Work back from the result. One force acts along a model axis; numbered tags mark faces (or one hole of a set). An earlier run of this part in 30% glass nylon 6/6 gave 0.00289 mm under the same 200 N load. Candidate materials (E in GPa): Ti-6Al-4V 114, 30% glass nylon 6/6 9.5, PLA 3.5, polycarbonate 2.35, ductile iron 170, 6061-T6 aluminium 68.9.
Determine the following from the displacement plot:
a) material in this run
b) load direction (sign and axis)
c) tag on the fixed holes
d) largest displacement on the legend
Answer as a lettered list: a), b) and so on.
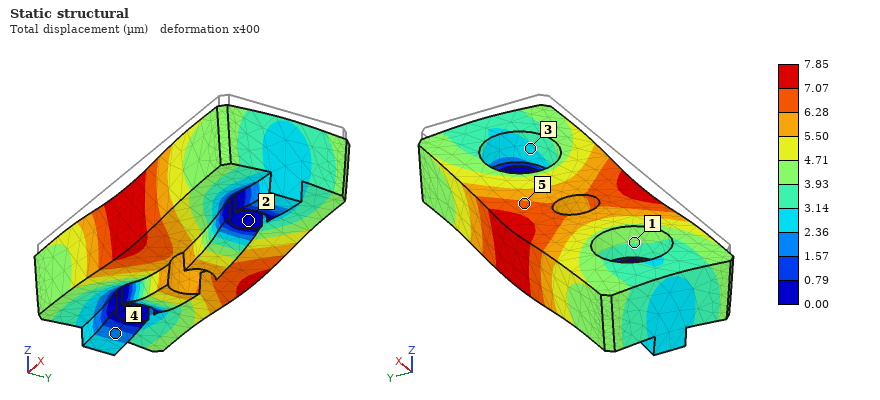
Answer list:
a) PLA
b) -Z
c) 2
d) 7.85 µm
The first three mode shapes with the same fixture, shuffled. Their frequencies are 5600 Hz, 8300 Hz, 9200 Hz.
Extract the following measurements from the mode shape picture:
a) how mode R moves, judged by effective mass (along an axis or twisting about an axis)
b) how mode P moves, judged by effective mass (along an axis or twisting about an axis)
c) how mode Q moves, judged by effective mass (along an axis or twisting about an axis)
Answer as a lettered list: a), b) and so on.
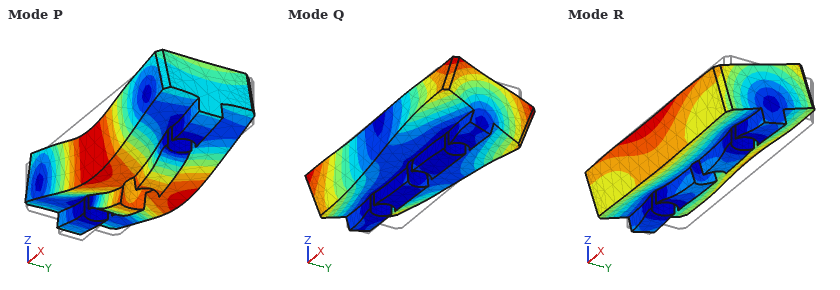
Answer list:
a) along Y
b) along Z
c) twisting about Z
